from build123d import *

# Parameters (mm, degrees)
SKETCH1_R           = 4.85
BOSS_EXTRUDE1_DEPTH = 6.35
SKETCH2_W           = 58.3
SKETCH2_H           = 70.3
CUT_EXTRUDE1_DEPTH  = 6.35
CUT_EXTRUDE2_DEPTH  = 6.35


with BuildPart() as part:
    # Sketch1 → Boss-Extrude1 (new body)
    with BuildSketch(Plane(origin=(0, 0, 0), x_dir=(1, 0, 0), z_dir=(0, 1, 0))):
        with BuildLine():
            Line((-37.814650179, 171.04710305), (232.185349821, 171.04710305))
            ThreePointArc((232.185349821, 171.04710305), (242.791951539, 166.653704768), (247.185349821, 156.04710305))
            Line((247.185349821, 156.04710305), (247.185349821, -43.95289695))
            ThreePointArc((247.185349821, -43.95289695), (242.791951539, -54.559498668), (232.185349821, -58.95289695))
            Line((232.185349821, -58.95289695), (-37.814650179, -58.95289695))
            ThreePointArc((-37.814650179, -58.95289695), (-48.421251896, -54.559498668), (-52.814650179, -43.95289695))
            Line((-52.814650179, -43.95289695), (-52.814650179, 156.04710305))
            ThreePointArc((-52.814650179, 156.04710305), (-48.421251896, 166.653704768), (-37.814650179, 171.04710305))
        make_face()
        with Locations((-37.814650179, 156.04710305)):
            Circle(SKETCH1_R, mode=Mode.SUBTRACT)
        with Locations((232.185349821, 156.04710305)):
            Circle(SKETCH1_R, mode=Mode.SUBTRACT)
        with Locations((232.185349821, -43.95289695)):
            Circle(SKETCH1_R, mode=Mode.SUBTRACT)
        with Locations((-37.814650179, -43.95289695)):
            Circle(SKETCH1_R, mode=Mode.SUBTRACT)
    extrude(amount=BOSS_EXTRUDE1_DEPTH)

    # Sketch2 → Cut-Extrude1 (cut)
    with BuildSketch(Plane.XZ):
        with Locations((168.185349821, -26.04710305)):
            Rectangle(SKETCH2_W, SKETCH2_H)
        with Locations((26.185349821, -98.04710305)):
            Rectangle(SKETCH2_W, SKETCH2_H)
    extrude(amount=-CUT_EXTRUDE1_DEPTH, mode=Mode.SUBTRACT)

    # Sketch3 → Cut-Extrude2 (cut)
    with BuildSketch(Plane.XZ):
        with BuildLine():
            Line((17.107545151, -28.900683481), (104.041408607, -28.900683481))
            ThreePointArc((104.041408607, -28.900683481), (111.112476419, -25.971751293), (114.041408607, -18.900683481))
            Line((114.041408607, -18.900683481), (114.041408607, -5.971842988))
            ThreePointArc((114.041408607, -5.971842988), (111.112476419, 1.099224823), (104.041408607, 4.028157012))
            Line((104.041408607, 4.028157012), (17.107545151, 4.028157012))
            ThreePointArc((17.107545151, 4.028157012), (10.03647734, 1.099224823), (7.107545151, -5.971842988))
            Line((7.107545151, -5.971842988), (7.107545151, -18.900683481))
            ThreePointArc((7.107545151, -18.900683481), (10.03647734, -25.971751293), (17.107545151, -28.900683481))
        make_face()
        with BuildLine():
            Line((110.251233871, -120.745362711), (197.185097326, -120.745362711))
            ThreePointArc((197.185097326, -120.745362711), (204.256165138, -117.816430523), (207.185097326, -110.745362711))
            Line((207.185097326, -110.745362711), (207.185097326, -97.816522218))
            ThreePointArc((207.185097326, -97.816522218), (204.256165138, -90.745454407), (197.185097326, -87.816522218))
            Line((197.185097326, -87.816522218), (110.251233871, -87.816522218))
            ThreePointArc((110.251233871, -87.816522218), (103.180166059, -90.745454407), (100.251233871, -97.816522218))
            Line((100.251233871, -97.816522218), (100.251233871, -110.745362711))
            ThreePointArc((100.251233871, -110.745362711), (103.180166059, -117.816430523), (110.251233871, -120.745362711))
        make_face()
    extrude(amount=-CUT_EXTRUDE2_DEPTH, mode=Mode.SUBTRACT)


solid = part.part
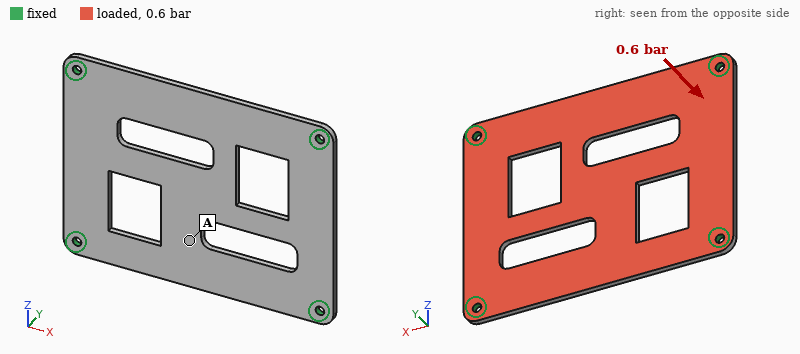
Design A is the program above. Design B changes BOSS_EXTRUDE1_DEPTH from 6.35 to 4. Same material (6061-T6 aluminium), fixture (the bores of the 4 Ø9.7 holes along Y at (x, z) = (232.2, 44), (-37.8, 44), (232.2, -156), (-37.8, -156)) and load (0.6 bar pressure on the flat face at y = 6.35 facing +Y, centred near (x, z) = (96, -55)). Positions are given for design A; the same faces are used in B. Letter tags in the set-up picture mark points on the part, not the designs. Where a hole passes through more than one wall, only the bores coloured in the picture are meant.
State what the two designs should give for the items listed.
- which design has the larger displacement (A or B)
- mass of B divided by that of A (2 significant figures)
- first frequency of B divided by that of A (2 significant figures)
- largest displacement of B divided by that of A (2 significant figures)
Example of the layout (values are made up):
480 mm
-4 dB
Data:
B
0.63
0.64
3.8
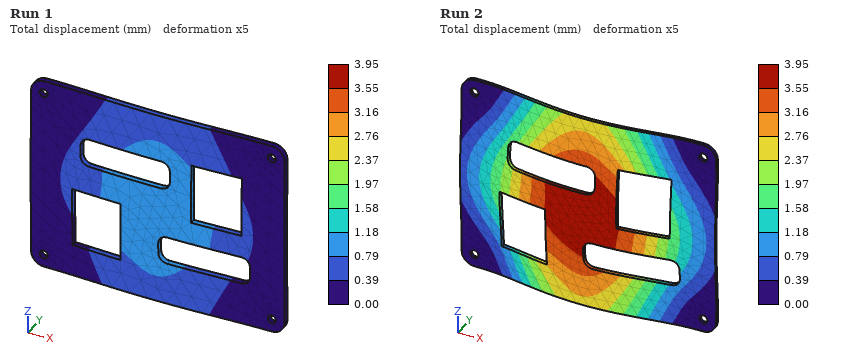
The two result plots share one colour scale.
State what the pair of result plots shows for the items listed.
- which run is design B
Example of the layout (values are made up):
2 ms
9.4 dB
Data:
Run 2
